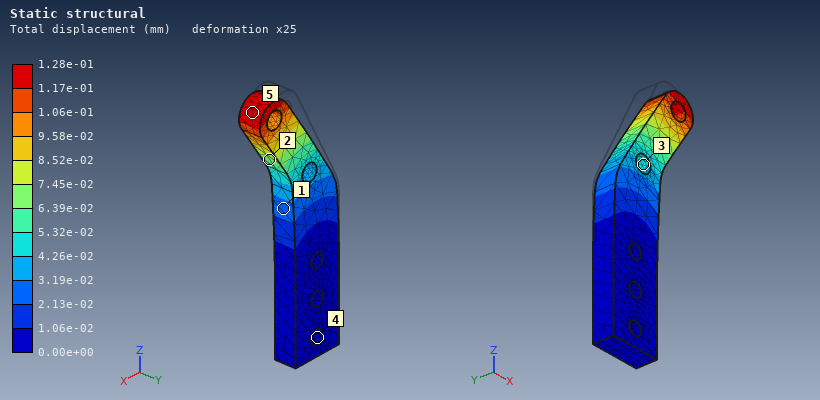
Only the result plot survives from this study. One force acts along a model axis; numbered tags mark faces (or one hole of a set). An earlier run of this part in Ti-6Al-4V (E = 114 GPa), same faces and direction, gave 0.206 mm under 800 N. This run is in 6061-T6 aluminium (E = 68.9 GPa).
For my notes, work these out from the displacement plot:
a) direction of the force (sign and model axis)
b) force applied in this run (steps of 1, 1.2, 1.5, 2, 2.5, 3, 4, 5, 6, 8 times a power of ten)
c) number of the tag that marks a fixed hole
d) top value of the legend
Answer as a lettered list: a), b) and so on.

a) +X
b) 300 N
c) 4
d) 1.28e-01 mm
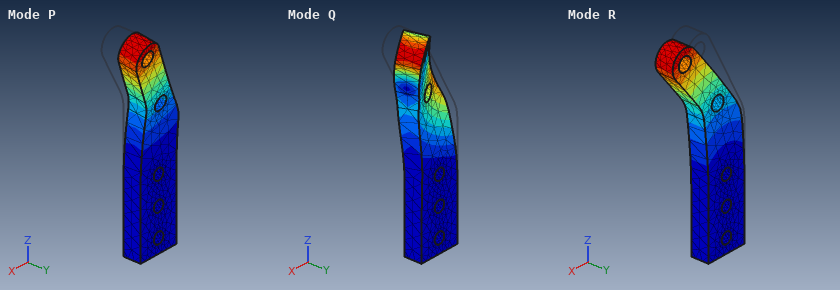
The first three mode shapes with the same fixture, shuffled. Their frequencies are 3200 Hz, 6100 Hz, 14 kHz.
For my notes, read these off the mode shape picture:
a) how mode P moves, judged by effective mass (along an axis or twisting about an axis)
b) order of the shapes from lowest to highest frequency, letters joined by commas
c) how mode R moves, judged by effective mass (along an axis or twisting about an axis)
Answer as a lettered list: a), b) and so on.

a) along Y
b) P, R, Q
c) along X
